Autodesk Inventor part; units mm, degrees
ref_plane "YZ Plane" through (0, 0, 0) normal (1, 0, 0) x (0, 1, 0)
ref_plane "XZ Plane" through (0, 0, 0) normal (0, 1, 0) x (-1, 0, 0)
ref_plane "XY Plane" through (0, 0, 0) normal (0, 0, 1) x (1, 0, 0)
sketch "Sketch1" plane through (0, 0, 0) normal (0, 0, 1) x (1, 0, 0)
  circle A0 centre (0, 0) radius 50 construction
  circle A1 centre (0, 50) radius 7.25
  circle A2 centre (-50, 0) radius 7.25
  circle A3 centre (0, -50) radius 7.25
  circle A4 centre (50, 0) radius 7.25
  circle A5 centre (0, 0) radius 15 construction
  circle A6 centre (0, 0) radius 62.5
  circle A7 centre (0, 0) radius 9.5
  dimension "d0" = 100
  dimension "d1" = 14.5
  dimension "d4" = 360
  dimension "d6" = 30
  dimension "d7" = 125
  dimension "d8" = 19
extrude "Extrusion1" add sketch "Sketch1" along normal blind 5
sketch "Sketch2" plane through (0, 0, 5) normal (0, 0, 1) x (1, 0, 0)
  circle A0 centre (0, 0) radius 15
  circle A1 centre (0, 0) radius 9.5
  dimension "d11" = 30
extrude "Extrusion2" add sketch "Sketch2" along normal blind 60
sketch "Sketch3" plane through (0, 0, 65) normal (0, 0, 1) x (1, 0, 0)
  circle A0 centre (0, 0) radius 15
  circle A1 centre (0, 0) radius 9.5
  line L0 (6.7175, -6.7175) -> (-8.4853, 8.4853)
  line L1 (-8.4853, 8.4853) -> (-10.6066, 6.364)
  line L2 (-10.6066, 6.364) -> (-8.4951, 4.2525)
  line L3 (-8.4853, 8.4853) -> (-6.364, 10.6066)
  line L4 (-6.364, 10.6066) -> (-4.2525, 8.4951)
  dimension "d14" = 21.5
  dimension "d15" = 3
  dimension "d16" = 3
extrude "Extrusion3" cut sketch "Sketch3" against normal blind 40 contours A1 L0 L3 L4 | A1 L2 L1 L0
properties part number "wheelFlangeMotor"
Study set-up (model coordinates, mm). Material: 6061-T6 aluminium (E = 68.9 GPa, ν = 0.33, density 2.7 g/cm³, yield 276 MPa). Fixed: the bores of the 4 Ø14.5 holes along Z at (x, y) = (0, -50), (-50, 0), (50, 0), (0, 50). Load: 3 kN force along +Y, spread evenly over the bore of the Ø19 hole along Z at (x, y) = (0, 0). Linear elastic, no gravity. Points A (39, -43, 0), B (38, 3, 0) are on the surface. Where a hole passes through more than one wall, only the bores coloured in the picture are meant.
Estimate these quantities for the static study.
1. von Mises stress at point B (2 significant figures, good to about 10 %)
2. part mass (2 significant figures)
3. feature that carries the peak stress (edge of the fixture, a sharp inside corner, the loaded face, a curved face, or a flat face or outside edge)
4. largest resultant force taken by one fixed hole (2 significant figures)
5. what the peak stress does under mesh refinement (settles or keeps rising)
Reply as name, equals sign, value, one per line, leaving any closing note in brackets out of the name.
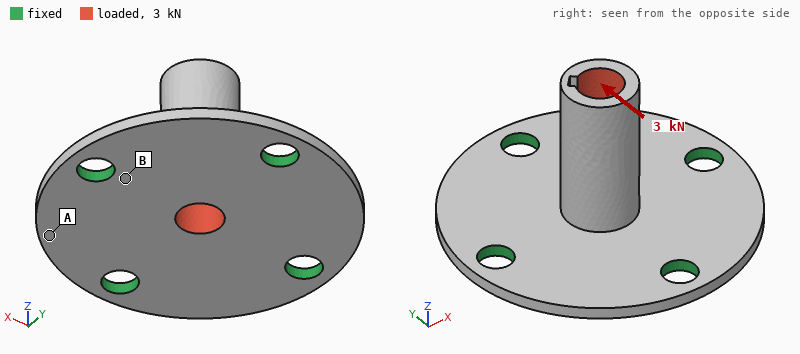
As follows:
von Mises stress at point B = 24 MPa
part mass = 220 g
feature that carries the peak stress = edge of the fixture
largest resultant force taken by one fixed hole = 1.6 kN
what the peak stress does under mesh refinement = keeps rising
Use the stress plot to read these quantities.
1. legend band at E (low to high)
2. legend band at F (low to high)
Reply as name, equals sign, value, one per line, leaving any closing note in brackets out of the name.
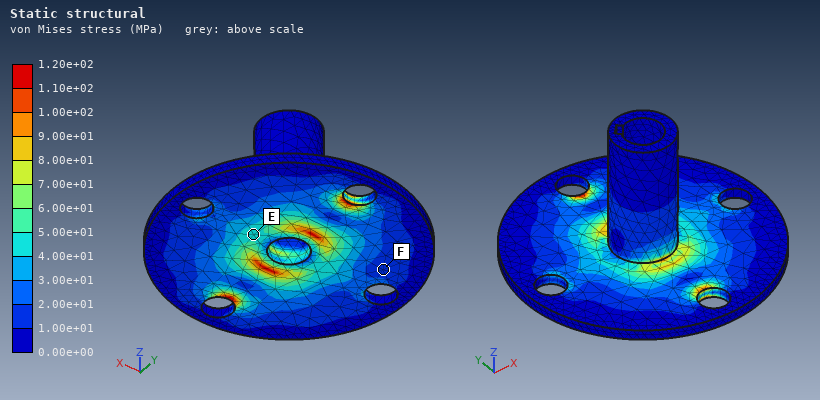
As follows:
legend band at E = 4.00e+01 to 5.00e+01 MPa
legend band at F = 1.00e+01 to 2.00e+01 MPa
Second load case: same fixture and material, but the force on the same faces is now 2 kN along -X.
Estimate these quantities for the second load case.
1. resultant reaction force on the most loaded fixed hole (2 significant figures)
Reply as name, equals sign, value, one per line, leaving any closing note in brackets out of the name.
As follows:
resultant reaction force on the most loaded fixed hole = 1.1 kN
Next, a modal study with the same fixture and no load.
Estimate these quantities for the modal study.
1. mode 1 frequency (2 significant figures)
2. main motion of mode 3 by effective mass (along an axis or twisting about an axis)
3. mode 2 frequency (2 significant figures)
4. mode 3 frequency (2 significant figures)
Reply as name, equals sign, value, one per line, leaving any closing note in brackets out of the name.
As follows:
mode 1 frequency = 2000 Hz
main motion of mode 3 by effective mass = along Z
mode 2 frequency = 2000 Hz
mode 3 frequency = 3000 Hz
